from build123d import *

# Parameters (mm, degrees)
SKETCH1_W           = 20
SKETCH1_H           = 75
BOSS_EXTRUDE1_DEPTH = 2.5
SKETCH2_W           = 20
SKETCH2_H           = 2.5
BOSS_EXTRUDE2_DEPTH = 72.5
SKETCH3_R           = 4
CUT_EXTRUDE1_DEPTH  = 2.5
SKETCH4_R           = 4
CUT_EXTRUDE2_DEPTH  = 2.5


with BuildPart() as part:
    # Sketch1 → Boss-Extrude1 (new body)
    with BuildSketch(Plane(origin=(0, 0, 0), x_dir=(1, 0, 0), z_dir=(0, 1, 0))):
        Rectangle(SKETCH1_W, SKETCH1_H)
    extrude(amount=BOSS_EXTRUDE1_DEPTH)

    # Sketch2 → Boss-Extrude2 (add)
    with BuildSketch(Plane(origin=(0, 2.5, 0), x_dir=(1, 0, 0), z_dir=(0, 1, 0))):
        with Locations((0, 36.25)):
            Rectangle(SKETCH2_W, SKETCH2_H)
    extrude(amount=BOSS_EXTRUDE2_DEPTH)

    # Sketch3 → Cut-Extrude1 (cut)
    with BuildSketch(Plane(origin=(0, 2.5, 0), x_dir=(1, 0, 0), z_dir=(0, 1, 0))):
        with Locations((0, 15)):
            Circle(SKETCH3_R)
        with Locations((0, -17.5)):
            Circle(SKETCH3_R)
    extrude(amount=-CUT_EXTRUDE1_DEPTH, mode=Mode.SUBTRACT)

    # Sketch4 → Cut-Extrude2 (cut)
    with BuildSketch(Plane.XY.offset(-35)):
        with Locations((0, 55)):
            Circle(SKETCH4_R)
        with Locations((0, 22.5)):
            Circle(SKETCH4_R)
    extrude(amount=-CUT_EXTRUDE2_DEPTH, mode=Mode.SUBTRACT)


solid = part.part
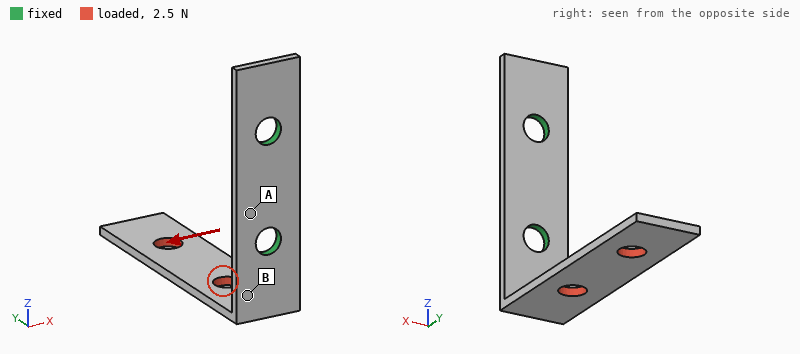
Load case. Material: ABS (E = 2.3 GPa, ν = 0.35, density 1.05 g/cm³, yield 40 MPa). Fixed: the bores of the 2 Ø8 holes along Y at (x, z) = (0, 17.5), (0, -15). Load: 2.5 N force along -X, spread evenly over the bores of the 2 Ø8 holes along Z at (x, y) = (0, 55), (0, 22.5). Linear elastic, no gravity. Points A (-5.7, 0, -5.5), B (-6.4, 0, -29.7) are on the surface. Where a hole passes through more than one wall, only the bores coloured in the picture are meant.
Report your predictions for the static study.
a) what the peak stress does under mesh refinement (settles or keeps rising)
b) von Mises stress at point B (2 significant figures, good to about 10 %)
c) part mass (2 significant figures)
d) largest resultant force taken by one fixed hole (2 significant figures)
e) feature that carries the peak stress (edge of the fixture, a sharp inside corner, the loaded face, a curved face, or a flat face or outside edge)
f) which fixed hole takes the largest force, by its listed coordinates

keeps rising
3.0 MPa
7.2 g
3.0 N
edge of the fixture
(0, -15)
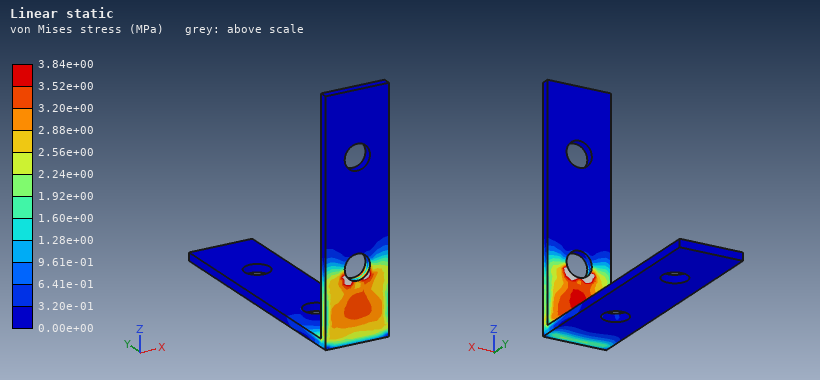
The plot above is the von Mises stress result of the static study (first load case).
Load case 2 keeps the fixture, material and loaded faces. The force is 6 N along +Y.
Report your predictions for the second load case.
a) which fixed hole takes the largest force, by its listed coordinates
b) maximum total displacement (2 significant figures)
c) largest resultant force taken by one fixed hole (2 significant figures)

(0, -15)
1.2 mm
6.0 N
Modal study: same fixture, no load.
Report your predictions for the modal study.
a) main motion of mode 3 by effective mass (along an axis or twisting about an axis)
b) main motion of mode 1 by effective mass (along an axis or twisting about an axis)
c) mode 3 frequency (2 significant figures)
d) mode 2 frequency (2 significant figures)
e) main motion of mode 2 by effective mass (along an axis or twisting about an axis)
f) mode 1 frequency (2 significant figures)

along Y
along Z
450 Hz
150 Hz
along X
80 Hz
